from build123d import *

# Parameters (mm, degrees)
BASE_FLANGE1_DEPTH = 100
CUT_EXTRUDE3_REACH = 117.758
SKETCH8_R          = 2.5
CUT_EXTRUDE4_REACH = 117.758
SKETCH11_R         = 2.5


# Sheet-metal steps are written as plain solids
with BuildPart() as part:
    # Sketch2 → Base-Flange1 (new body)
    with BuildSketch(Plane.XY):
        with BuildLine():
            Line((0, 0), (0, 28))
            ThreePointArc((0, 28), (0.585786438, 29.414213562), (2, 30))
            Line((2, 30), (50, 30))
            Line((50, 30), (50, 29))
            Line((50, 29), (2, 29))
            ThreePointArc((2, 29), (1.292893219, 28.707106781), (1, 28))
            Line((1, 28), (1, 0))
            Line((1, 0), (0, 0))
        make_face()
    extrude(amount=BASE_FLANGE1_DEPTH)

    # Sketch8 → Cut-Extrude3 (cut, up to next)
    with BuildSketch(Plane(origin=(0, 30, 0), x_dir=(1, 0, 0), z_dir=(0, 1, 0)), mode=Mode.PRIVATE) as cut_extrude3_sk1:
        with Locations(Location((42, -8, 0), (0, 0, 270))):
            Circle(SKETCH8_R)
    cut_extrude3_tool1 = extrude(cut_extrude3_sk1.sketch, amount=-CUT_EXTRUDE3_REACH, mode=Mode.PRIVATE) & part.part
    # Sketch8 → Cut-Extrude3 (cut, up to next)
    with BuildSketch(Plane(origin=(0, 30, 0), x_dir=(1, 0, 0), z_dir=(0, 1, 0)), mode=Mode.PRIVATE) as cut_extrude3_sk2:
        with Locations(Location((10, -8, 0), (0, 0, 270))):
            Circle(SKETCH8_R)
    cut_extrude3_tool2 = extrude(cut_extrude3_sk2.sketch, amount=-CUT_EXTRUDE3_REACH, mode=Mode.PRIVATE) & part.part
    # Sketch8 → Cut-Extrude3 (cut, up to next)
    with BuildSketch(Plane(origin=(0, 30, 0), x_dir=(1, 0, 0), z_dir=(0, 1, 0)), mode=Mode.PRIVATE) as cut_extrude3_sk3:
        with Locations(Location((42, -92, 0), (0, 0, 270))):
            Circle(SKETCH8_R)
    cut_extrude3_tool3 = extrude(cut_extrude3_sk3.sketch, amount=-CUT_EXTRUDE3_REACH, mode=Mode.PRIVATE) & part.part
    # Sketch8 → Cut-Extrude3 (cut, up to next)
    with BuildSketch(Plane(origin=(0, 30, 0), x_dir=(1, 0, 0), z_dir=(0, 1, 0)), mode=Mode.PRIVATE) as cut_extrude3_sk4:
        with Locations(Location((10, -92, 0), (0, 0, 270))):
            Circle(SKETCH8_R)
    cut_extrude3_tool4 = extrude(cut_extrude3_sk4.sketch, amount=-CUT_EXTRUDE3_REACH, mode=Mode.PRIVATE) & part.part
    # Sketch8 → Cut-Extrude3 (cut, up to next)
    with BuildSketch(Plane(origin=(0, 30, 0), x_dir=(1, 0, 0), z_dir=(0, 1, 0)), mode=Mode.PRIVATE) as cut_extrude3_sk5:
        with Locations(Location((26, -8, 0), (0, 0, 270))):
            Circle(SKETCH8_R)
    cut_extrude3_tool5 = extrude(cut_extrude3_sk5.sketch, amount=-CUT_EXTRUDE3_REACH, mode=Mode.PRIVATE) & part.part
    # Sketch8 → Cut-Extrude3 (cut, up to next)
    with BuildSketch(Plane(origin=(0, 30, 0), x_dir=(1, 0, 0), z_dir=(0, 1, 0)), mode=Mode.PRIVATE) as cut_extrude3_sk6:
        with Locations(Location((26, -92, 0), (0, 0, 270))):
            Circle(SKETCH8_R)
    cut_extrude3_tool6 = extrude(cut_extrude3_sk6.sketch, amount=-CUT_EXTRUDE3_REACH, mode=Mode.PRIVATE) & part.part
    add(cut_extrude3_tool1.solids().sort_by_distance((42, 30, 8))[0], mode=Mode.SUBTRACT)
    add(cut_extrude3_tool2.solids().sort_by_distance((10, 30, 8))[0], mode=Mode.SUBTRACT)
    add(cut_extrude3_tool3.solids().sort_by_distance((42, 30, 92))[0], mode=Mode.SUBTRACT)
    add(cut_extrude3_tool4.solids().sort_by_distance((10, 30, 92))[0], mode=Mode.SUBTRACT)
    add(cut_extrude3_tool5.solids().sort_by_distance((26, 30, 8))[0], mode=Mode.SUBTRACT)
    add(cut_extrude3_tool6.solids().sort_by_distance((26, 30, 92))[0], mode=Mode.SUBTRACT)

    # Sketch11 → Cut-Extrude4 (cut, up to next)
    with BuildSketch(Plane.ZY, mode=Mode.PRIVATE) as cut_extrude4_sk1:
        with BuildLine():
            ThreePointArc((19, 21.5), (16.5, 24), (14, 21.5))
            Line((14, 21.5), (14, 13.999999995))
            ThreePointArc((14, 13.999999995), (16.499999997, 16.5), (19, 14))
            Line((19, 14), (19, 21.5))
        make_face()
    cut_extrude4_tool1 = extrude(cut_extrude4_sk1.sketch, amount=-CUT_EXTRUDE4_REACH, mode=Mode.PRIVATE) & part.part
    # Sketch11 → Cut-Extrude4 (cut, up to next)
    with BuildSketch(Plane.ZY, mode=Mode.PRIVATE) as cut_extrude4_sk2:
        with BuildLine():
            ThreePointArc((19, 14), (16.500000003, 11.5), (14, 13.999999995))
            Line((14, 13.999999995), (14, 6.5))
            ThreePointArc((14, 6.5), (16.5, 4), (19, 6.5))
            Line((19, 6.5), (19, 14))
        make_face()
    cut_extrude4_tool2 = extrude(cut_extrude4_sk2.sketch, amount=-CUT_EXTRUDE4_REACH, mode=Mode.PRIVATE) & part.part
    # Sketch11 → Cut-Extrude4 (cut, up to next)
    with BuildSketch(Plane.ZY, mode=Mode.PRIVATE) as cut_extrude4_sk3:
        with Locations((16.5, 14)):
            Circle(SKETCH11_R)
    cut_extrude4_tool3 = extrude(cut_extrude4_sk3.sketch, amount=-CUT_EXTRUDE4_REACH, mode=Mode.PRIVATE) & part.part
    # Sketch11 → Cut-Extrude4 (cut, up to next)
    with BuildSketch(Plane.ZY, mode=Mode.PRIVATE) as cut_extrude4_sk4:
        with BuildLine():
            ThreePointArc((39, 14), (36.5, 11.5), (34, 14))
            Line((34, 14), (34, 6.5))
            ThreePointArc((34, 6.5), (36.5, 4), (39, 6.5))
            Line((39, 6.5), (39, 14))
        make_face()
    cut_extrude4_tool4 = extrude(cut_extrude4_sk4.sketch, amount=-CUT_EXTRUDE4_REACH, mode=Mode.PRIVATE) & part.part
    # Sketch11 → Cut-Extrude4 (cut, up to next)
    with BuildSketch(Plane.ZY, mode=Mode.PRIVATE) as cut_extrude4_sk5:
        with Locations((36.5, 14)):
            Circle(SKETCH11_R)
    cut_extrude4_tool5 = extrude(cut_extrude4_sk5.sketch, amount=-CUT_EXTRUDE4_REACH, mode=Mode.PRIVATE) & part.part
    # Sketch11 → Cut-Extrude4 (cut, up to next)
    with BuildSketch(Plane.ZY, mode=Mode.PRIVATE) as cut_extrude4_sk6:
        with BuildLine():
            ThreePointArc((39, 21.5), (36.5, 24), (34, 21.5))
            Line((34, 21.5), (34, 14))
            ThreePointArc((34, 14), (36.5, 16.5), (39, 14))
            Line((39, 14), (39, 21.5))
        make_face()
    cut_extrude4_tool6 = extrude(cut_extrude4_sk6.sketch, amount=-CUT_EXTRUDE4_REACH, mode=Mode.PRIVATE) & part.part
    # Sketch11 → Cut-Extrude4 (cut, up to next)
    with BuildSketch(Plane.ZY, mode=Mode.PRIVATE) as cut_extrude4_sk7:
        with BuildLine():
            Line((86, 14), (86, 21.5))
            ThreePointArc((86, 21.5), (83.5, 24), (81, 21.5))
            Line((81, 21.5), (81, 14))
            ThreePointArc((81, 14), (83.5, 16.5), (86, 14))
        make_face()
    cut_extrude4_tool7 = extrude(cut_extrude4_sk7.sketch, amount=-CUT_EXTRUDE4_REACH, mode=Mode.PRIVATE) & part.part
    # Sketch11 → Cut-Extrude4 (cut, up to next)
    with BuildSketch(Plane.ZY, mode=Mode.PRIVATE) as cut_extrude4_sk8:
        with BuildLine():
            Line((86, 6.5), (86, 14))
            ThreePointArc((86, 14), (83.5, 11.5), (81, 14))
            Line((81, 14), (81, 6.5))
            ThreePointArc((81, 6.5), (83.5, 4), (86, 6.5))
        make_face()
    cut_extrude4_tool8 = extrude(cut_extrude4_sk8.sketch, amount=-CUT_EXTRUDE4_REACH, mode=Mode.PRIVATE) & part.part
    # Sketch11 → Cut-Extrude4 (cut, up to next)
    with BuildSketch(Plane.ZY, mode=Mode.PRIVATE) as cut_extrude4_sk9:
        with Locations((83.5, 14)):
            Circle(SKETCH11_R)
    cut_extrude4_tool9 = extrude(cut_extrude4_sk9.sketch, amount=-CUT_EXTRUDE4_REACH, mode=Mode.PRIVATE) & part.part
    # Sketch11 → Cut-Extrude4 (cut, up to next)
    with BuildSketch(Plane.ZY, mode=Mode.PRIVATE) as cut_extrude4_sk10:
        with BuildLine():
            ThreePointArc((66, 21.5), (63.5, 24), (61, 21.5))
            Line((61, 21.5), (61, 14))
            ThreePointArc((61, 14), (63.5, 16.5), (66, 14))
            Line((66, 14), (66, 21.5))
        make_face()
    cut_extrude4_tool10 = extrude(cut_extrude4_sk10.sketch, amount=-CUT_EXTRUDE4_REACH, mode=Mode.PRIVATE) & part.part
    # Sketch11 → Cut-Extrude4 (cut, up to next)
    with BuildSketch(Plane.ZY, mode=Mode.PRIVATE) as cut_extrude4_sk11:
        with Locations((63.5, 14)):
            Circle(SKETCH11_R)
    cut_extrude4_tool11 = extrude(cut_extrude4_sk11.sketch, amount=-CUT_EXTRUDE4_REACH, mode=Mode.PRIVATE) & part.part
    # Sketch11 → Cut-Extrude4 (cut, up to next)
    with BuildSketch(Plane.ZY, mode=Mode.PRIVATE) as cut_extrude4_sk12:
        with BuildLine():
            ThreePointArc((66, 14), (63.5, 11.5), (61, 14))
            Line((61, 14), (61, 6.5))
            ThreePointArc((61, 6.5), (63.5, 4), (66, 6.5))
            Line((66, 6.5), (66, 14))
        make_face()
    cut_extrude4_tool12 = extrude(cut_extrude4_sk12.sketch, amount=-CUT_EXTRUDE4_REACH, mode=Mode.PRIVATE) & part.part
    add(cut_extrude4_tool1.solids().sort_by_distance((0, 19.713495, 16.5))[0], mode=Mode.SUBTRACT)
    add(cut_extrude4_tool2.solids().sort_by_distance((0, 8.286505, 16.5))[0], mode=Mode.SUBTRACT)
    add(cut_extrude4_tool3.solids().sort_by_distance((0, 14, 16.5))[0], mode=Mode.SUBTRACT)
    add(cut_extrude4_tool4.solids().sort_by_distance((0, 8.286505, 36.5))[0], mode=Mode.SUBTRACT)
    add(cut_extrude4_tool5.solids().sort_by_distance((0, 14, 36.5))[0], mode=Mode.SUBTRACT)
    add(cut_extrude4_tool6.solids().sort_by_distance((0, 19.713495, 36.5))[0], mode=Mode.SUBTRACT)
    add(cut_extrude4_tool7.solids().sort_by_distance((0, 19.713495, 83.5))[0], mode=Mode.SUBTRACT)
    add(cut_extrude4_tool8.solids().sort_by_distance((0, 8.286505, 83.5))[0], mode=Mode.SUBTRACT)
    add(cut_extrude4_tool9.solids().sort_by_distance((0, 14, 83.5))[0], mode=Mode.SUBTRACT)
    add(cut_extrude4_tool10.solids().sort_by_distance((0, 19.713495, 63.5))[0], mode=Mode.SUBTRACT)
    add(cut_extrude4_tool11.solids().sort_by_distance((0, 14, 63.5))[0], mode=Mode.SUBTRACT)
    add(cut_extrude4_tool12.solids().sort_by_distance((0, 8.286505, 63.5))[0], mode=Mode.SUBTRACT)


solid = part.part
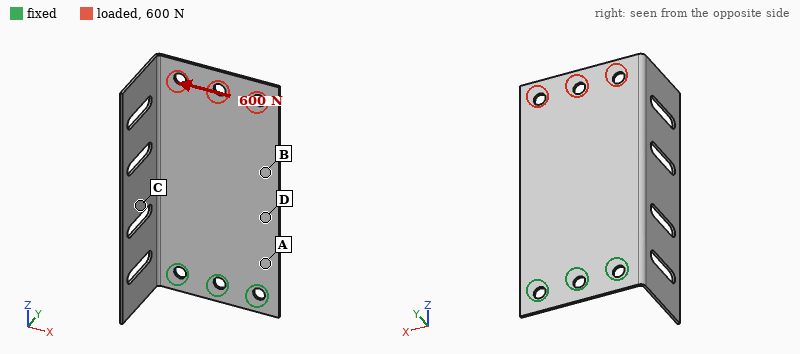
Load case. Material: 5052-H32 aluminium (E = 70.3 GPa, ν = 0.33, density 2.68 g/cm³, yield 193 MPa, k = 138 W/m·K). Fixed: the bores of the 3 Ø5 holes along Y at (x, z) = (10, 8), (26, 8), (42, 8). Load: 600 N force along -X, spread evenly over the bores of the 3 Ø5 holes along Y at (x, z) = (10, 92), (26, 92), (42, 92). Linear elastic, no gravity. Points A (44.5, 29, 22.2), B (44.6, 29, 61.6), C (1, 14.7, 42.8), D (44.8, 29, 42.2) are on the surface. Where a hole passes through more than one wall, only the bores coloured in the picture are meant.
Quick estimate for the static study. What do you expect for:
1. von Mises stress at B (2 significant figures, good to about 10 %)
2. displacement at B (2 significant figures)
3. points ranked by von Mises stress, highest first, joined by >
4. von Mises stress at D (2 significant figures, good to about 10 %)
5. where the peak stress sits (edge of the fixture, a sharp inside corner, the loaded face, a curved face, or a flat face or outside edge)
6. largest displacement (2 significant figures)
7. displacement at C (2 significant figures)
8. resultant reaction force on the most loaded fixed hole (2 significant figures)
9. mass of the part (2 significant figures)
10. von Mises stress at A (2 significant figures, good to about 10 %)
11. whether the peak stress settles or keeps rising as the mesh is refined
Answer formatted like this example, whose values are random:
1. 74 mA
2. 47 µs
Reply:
1. 34 MPa
2. 0.13 mm
3. A > D > B > C
4. 55 MPa
5. edge of the fixture
6. 0.28 mm
7. 0.076 mm
8. 1.5 kN
9. 20 g
10. 80 MPa
11. keeps rising
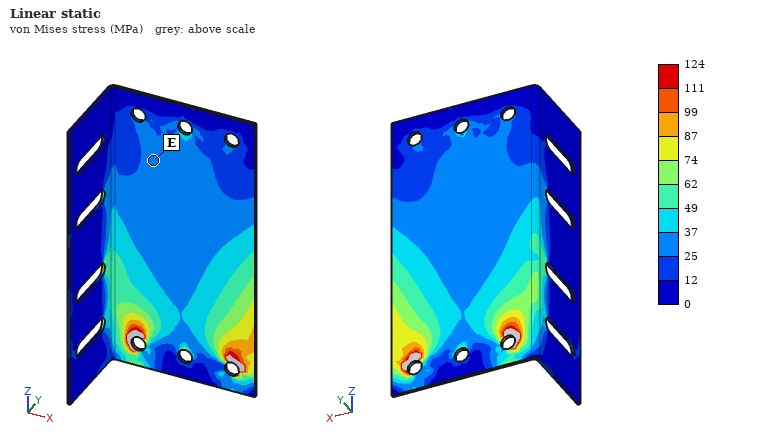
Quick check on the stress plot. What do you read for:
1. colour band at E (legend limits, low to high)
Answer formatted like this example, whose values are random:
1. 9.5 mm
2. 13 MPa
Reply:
1. 25 to 37 MPa
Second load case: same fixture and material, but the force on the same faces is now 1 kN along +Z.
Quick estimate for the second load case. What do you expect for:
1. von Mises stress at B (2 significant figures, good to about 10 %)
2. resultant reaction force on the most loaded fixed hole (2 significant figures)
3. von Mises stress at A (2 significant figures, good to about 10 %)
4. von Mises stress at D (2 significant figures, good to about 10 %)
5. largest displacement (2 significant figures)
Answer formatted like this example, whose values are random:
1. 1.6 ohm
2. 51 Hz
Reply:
1. 22 MPa
2. 360 N
3. 22 MPa
4. 22 MPa
5. 41 µm
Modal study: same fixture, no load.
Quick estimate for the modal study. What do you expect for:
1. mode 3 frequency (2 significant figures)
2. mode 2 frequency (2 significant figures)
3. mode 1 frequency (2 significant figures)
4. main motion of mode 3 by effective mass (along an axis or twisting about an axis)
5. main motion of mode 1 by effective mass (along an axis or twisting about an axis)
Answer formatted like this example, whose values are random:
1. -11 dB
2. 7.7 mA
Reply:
1. 710 Hz
2. 290 Hz
3. 160 Hz
4. along X
5. along Y
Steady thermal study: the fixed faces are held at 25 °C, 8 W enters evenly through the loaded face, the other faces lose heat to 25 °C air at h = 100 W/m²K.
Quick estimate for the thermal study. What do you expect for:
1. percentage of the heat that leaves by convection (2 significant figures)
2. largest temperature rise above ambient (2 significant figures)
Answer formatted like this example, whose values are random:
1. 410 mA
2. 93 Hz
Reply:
1. 95 %
2. 25 K
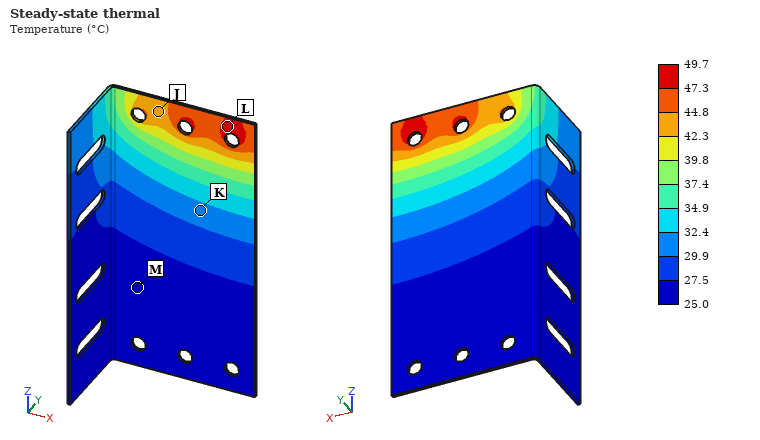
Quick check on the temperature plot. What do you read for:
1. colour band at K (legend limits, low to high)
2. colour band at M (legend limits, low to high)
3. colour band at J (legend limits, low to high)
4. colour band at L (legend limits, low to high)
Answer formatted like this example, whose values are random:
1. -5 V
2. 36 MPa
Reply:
1. 29.9 to 32.4 °C
2. 25.0 to 27.5 °C
3. 42.3 to 44.8 °C
4. 47.3 to 49.7 °C
